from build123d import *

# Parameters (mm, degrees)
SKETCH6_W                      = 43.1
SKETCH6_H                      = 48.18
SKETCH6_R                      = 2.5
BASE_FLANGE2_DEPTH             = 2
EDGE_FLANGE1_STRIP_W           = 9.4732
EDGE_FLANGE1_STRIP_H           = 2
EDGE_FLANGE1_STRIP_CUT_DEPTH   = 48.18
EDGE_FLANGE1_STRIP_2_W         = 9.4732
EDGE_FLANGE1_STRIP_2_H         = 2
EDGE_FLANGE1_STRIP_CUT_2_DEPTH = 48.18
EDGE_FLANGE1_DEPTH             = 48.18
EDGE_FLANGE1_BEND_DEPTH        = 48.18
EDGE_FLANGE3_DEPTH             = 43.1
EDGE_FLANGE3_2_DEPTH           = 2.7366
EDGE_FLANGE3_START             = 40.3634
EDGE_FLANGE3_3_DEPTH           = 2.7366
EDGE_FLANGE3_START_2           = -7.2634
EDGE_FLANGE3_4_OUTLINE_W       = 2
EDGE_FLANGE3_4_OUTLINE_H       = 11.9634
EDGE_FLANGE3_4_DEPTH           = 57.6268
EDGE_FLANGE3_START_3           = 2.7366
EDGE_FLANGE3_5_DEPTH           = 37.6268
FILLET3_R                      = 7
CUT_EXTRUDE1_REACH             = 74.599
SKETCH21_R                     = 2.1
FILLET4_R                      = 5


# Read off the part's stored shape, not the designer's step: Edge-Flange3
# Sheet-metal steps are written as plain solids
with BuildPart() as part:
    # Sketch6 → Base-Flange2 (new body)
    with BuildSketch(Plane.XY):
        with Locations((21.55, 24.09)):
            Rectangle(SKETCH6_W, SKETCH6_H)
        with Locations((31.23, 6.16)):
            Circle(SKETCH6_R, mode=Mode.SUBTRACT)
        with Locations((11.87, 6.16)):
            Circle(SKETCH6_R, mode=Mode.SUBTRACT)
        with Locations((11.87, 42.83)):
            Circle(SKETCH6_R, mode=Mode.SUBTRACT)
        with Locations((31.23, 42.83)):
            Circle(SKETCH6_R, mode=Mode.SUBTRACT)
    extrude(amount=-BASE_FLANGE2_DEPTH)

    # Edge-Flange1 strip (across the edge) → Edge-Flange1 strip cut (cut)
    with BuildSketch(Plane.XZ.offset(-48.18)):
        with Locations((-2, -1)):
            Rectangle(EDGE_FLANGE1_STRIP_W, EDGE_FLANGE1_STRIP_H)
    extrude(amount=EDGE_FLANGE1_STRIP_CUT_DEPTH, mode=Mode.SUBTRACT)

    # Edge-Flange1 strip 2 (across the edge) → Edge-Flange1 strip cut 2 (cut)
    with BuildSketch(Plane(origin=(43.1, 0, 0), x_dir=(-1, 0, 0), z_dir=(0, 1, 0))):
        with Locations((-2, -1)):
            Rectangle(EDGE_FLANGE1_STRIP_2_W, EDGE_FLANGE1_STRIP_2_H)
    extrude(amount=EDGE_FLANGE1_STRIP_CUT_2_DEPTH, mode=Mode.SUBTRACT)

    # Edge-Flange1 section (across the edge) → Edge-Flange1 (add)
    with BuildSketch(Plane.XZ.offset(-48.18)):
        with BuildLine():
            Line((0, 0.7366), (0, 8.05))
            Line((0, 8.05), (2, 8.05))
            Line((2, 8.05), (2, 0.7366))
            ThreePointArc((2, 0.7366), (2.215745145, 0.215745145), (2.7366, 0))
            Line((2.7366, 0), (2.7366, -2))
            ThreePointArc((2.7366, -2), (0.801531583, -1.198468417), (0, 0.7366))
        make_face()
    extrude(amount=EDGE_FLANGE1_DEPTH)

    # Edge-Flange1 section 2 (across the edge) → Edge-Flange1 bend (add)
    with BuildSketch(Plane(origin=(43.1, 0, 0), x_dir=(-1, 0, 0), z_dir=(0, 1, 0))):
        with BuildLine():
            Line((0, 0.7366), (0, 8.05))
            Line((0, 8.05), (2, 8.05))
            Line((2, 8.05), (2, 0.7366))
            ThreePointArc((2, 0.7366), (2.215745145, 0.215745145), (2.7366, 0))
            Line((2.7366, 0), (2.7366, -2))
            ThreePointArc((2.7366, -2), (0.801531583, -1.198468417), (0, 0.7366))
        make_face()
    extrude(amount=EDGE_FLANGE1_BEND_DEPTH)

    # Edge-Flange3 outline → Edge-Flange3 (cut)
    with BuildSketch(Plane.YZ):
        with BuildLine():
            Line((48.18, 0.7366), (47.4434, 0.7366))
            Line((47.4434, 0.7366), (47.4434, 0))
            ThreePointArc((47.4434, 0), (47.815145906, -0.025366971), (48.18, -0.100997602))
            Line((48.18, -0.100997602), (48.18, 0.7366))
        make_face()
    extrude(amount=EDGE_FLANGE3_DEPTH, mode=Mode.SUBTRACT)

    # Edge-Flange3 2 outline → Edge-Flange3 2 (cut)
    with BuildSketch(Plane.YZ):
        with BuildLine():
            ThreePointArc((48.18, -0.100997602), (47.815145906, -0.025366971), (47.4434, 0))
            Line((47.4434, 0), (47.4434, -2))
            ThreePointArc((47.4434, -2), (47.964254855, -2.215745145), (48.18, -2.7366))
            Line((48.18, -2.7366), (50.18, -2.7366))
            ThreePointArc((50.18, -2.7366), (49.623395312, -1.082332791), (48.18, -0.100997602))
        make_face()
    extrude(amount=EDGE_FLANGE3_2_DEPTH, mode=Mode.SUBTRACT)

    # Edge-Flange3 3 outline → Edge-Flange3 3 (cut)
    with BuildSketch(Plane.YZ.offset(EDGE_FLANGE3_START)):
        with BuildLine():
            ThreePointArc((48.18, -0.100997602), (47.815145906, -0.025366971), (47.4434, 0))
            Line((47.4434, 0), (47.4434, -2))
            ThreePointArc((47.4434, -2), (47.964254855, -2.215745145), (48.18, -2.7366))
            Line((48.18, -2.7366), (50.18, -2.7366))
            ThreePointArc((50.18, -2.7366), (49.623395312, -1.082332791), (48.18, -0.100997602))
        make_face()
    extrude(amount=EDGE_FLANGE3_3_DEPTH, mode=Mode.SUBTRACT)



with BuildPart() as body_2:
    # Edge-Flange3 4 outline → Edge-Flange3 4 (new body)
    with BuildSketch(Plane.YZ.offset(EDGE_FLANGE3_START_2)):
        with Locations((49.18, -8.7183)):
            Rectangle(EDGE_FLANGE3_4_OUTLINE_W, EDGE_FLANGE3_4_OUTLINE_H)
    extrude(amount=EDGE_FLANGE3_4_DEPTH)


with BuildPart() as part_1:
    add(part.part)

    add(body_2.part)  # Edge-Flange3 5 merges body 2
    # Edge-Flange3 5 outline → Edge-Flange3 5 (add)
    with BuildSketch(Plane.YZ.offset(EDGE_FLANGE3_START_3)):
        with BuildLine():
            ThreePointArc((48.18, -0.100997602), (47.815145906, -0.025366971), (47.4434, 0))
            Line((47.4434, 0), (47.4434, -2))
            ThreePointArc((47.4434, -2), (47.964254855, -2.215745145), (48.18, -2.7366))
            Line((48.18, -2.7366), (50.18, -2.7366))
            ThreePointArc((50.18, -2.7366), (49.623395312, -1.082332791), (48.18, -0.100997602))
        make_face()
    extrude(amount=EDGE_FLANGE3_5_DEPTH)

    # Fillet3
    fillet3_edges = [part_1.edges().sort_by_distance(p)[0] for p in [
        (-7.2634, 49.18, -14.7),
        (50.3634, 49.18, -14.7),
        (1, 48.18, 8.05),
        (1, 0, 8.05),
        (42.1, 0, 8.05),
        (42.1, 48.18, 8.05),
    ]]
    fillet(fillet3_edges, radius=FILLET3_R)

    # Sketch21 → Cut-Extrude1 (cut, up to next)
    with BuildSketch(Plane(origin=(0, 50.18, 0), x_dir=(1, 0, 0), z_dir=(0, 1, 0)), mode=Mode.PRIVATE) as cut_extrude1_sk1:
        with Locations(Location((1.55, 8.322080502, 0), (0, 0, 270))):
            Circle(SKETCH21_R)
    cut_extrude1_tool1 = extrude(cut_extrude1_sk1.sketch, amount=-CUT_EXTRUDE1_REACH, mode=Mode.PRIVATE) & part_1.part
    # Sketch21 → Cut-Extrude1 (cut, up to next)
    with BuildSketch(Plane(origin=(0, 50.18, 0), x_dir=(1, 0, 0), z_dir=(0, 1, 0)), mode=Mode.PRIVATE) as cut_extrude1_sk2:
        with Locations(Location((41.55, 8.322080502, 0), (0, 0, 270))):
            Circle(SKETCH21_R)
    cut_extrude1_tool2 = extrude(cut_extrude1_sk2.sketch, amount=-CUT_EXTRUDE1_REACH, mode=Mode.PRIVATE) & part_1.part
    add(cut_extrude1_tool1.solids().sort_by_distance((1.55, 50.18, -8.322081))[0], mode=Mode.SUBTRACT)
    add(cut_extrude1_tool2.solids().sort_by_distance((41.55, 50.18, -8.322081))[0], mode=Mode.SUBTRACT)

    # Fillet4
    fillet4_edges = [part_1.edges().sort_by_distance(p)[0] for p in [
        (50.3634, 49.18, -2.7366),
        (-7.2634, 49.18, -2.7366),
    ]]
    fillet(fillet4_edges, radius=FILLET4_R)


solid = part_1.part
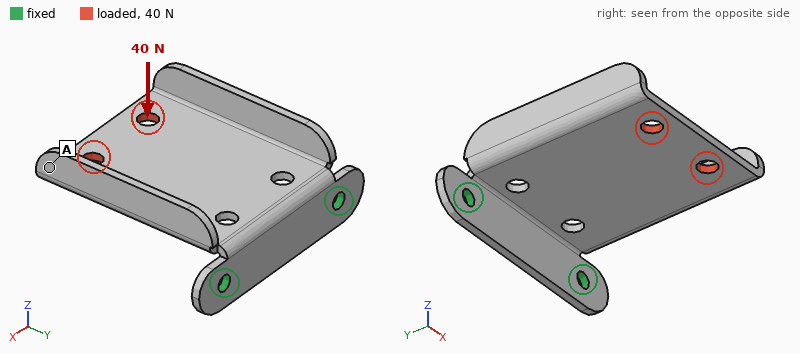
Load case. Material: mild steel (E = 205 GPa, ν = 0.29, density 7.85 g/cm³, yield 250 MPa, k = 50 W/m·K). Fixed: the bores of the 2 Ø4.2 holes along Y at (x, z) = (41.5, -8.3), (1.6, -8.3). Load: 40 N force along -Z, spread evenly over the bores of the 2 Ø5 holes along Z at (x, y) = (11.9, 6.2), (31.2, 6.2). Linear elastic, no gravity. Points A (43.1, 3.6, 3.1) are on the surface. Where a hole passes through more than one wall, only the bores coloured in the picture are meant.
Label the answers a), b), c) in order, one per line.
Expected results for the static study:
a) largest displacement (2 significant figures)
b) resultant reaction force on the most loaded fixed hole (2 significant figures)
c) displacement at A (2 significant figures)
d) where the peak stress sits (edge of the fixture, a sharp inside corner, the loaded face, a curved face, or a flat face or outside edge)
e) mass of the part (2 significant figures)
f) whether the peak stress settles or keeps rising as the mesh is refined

a) 0.26 mm
b) 27 N
c) 0.23 mm
d) a sharp inside corner
e) 53 g
f) keeps rising
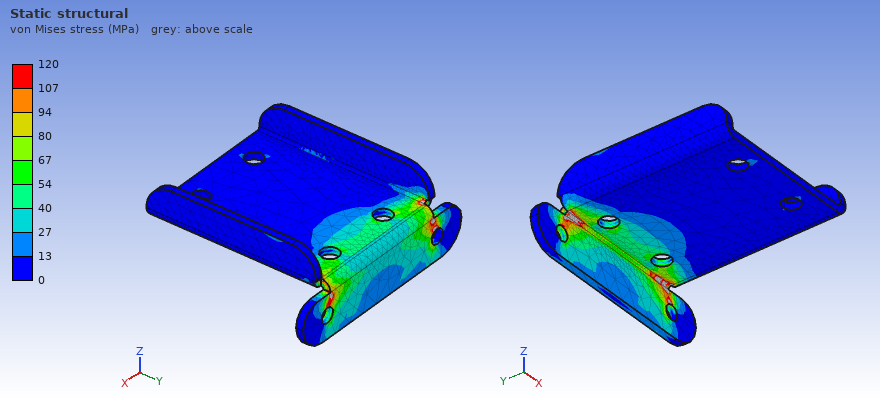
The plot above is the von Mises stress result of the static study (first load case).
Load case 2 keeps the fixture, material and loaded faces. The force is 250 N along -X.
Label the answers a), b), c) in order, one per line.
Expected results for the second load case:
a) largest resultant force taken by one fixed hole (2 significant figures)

a) 330 N
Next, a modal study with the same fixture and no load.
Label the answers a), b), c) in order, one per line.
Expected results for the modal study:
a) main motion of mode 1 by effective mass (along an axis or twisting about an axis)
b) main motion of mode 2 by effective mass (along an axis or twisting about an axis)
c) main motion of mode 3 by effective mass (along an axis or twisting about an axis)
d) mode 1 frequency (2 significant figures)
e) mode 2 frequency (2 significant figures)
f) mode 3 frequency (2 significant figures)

a) along Z
b) twisting about Y
c) along X
d) 500 Hz
e) 1300 Hz
f) 2800 Hz
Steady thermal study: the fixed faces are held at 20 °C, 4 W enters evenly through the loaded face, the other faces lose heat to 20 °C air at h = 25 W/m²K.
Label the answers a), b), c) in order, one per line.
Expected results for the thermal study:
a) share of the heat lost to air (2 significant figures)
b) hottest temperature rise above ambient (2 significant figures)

a) 61 %
b) 30 K
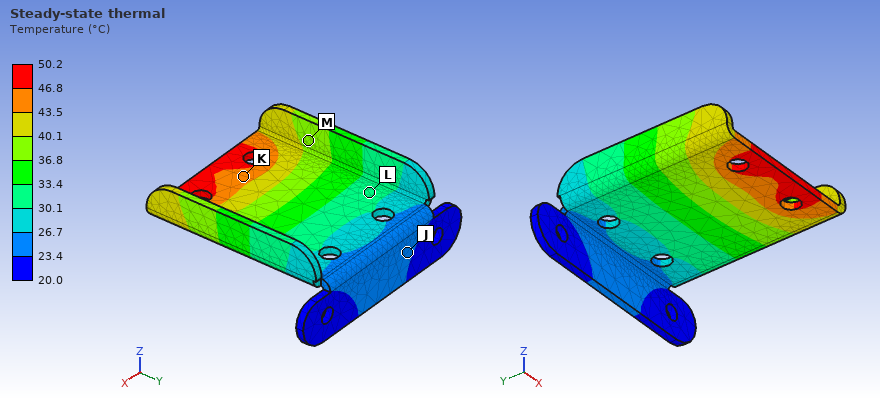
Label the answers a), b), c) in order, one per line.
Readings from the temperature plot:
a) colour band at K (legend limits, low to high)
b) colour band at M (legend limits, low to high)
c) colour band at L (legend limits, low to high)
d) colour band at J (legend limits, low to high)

a) 43.5 to 46.8 °C
b) 36.8 to 40.1 °C
c) 30.1 to 33.4 °C
d) 23.4 to 26.7 °C
